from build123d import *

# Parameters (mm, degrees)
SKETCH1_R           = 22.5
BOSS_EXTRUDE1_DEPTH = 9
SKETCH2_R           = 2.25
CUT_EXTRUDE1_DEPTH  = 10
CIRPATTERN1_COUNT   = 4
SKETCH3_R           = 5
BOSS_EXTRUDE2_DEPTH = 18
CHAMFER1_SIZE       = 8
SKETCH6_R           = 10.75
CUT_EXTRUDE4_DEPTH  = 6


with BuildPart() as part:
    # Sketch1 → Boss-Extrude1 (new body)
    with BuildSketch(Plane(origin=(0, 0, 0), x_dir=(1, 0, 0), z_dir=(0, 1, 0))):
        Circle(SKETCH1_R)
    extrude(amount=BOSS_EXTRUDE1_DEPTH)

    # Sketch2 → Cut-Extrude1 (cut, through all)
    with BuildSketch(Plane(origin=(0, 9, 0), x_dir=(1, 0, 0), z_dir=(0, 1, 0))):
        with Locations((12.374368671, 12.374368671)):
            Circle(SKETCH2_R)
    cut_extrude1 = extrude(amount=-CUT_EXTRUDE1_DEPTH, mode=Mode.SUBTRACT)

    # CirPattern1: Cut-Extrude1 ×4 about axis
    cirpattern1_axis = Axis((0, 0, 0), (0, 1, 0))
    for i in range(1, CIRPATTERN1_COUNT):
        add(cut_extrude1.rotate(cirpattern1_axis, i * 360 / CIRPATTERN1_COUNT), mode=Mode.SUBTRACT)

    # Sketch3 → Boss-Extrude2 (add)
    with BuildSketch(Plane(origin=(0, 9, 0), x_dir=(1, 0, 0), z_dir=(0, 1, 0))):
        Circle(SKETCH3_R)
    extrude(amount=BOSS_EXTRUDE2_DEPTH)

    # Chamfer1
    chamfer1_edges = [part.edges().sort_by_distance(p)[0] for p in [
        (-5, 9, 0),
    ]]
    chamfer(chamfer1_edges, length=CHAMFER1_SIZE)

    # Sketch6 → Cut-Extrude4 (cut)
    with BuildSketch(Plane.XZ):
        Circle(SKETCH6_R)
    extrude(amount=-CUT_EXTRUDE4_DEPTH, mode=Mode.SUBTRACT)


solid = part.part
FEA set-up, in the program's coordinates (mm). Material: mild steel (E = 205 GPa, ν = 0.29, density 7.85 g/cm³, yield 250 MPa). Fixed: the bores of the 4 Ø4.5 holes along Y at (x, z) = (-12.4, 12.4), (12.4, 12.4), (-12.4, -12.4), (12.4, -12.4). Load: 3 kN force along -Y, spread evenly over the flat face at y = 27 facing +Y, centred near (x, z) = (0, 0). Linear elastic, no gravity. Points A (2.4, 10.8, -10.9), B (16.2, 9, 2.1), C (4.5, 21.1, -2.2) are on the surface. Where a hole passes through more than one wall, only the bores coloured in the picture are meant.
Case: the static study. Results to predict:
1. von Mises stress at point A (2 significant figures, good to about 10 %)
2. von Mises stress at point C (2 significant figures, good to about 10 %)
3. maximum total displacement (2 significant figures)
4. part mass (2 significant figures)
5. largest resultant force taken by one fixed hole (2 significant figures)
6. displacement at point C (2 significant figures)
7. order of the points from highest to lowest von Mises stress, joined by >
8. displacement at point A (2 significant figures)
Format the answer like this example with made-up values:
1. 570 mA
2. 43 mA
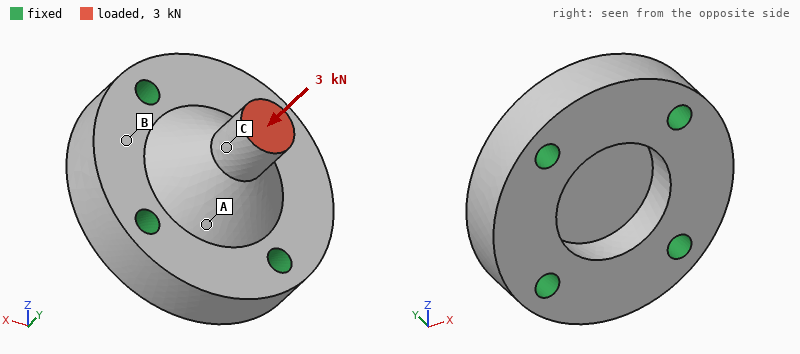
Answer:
1. 13 MPa
2. 37 MPa
3. 4.0 µm
4. 110 g
5. 870 N
6. 3.0 µm
7. C > A > B
8. 0.86 µm
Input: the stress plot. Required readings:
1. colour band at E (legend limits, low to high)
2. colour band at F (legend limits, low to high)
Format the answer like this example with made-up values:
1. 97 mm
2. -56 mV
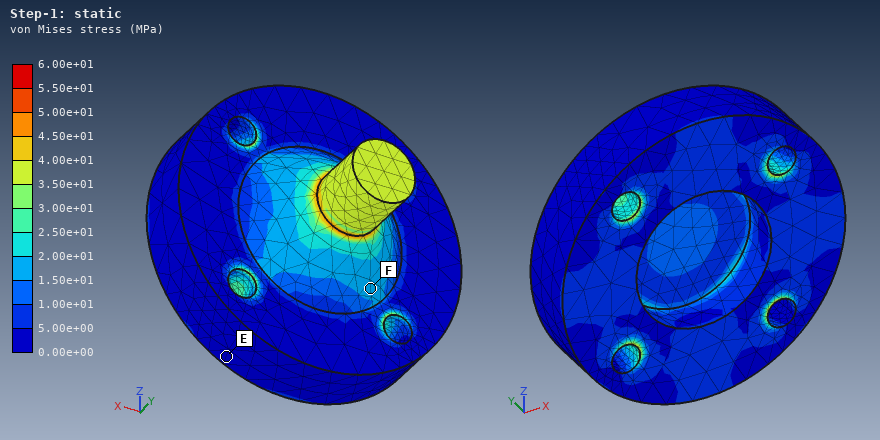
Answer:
1. 0.00e+00 to 5.00e+00 MPa
2. 1.50e+01 to 2.00e+01 MPa
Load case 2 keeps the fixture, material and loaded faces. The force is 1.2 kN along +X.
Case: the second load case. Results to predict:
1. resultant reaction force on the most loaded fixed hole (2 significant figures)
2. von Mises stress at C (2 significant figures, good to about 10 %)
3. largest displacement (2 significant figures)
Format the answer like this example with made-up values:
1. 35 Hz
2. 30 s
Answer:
1. 670 N
2. 65 MPa
3. 14 µm
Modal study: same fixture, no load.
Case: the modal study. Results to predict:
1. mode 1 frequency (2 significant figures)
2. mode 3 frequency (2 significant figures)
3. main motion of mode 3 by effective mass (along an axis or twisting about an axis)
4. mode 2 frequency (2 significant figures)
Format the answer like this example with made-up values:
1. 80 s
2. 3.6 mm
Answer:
1. 29 kHz
2. 37 kHz
3. along Y
4. 29 kHz
